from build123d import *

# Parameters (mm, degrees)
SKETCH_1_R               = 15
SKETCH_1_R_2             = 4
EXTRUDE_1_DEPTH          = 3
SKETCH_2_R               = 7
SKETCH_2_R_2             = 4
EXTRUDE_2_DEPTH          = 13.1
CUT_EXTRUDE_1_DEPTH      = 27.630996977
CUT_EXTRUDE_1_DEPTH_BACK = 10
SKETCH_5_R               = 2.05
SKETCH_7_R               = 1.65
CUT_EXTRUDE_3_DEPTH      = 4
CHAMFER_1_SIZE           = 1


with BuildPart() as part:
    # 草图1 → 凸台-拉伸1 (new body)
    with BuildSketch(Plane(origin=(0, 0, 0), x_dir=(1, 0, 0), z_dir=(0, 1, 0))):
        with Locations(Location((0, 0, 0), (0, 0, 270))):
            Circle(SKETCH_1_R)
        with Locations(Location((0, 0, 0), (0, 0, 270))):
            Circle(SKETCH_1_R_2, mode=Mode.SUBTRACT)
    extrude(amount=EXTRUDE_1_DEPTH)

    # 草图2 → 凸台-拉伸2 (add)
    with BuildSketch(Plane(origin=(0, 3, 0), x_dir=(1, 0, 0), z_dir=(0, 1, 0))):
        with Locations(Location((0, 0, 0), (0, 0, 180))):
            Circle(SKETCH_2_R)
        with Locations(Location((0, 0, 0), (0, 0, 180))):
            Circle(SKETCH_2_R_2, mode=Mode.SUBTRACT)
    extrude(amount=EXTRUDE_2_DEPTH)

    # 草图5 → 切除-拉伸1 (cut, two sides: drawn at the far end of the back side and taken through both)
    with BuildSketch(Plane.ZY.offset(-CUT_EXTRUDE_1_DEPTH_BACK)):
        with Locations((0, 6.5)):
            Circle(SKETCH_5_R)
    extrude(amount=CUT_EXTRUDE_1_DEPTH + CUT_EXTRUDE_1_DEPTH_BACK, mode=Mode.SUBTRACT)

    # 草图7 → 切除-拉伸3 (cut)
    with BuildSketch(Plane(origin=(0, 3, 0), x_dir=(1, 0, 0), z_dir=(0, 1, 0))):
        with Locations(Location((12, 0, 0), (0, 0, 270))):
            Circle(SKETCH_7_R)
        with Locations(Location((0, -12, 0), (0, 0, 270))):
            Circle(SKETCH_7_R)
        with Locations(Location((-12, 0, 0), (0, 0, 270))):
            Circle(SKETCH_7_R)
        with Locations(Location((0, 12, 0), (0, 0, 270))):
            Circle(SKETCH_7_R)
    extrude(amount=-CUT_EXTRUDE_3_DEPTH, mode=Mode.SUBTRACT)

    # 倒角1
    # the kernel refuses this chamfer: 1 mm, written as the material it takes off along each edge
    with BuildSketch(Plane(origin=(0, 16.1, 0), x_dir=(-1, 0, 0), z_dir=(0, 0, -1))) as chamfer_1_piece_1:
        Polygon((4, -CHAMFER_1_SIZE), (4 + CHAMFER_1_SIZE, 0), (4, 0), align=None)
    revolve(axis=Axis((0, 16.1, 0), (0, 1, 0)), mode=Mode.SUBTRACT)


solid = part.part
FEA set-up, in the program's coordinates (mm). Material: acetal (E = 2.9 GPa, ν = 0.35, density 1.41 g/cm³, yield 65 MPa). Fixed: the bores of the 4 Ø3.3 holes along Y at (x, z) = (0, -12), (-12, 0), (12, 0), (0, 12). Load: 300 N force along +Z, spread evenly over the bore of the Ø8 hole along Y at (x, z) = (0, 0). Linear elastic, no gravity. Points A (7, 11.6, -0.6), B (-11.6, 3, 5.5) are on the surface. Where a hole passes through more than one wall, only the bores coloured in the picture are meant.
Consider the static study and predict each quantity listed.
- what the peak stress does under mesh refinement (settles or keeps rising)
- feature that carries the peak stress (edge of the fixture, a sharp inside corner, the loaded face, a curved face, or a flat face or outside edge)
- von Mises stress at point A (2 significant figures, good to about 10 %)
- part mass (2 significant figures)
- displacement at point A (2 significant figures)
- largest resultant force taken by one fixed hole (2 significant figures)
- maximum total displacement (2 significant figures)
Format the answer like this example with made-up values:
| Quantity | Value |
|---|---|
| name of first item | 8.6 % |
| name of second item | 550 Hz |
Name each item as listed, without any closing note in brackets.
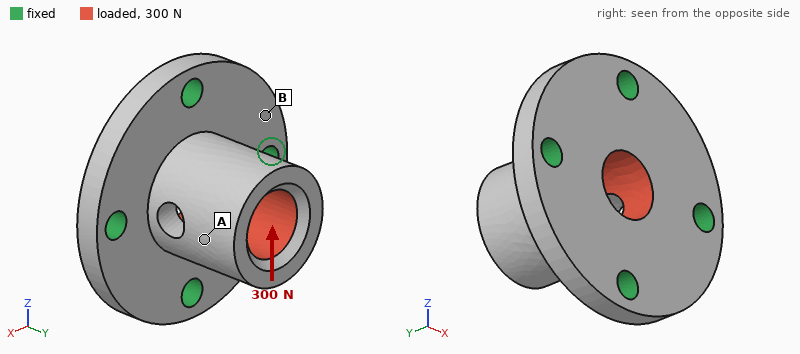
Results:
| Quantity | Value |
|---|---|
| what the peak stress does under mesh refinement | keeps rising |
| feature that carries the peak stress | edge of the fixture |
| von Mises stress at point A | 3.6 MPa |
| part mass | 4.4 g |
| displacement at point A | 0.080 mm |
| largest resultant force taken by one fixed hole | 130 N |
| maximum total displacement | 0.12 mm |
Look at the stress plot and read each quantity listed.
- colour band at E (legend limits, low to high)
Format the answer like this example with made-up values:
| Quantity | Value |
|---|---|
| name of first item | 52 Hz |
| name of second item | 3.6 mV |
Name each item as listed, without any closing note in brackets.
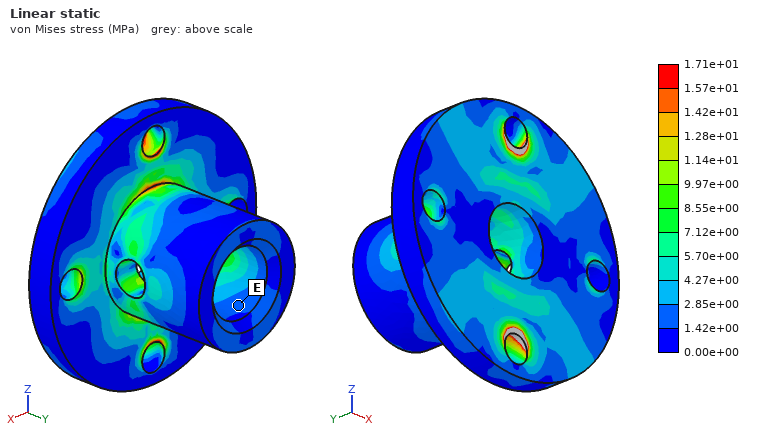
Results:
| Quantity | Value |
|---|---|
| colour band at E | 1.42e+00 to 2.85e+00 MPa |
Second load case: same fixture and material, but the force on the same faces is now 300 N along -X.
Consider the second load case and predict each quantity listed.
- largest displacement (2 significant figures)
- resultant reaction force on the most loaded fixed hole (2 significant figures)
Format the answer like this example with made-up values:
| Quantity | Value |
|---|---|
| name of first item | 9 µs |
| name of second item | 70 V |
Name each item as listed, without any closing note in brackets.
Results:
| Quantity | Value |
|---|---|
| largest displacement | 0.12 mm |
| resultant reaction force on the most loaded fixed hole | 130 N |
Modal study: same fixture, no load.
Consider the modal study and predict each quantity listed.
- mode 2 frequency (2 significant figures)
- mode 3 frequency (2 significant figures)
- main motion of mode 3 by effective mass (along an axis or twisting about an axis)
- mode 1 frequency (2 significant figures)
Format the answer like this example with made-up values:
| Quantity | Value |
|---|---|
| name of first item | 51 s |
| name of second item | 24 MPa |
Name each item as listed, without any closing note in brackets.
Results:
| Quantity | Value |
|---|---|
| mode 2 frequency | 5900 Hz |
| mode 3 frequency | 8700 Hz |
| main motion of mode 3 by effective mass | along Y |
| mode 1 frequency | 5800 Hz |
